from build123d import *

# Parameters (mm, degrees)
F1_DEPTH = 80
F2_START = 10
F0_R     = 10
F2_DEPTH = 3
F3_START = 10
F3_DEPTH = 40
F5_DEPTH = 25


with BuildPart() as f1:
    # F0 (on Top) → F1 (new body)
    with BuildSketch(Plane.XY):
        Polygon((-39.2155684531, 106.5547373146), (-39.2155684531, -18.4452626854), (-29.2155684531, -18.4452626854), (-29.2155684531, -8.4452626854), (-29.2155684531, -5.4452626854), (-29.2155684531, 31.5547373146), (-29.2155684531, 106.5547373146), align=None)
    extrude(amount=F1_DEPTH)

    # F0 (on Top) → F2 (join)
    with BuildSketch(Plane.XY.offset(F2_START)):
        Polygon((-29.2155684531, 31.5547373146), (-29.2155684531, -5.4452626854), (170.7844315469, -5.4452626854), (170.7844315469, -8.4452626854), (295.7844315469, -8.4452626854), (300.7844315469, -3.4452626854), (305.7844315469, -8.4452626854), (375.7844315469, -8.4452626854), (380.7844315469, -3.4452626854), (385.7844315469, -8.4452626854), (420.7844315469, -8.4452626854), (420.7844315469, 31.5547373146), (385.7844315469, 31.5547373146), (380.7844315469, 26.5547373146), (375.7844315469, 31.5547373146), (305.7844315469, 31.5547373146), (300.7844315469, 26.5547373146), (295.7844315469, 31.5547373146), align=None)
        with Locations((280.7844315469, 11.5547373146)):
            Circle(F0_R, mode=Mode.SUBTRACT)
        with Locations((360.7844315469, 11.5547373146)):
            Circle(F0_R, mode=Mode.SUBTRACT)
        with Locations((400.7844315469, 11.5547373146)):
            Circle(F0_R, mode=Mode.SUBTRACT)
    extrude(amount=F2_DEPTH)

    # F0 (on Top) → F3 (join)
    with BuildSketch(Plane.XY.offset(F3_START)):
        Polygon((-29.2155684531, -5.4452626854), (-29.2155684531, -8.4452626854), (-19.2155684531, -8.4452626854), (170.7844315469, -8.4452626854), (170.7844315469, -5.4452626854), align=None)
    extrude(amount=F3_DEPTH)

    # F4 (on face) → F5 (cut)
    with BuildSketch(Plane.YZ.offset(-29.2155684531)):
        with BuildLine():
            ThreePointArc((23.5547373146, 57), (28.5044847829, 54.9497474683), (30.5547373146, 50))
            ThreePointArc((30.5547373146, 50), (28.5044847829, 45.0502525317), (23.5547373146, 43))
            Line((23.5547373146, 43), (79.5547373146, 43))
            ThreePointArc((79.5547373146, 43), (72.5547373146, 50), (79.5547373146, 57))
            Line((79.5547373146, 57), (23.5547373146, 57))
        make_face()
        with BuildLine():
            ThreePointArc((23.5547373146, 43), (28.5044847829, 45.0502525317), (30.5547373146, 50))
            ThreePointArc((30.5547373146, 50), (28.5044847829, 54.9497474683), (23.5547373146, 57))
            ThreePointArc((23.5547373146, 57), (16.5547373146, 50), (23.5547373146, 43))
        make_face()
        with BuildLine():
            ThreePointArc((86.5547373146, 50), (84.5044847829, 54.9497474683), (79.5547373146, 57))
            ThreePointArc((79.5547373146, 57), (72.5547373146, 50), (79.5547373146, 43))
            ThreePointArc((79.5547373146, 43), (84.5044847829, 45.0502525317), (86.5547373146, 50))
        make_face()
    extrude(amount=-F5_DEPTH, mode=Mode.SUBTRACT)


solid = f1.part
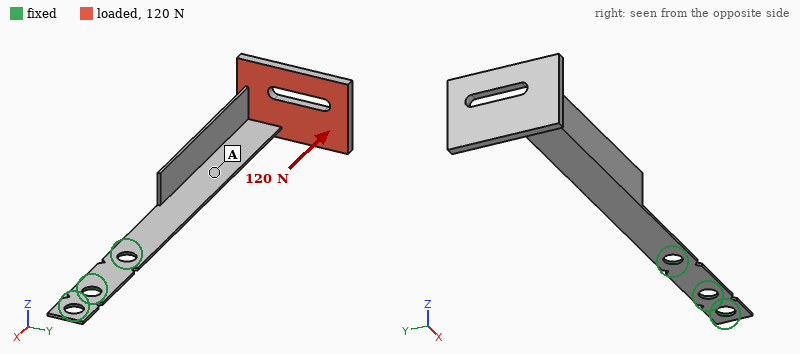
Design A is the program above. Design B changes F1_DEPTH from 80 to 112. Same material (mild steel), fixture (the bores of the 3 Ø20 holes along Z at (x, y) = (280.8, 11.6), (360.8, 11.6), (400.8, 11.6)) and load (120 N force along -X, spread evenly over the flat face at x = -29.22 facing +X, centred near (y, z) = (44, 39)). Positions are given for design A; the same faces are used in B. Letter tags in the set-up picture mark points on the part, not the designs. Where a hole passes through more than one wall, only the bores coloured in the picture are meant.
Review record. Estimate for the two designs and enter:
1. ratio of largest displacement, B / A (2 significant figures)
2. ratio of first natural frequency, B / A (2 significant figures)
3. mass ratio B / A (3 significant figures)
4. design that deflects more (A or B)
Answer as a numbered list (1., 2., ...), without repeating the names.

1. 1.7
2. 0.84
3. 1.24
4. B
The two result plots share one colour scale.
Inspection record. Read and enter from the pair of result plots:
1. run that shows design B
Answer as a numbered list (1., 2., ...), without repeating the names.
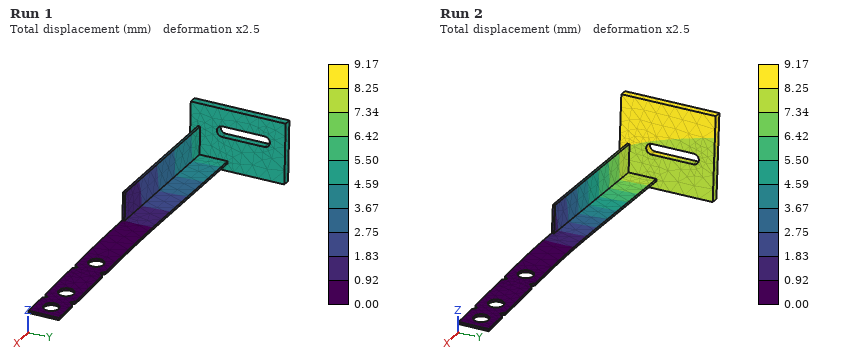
1. Run 2
